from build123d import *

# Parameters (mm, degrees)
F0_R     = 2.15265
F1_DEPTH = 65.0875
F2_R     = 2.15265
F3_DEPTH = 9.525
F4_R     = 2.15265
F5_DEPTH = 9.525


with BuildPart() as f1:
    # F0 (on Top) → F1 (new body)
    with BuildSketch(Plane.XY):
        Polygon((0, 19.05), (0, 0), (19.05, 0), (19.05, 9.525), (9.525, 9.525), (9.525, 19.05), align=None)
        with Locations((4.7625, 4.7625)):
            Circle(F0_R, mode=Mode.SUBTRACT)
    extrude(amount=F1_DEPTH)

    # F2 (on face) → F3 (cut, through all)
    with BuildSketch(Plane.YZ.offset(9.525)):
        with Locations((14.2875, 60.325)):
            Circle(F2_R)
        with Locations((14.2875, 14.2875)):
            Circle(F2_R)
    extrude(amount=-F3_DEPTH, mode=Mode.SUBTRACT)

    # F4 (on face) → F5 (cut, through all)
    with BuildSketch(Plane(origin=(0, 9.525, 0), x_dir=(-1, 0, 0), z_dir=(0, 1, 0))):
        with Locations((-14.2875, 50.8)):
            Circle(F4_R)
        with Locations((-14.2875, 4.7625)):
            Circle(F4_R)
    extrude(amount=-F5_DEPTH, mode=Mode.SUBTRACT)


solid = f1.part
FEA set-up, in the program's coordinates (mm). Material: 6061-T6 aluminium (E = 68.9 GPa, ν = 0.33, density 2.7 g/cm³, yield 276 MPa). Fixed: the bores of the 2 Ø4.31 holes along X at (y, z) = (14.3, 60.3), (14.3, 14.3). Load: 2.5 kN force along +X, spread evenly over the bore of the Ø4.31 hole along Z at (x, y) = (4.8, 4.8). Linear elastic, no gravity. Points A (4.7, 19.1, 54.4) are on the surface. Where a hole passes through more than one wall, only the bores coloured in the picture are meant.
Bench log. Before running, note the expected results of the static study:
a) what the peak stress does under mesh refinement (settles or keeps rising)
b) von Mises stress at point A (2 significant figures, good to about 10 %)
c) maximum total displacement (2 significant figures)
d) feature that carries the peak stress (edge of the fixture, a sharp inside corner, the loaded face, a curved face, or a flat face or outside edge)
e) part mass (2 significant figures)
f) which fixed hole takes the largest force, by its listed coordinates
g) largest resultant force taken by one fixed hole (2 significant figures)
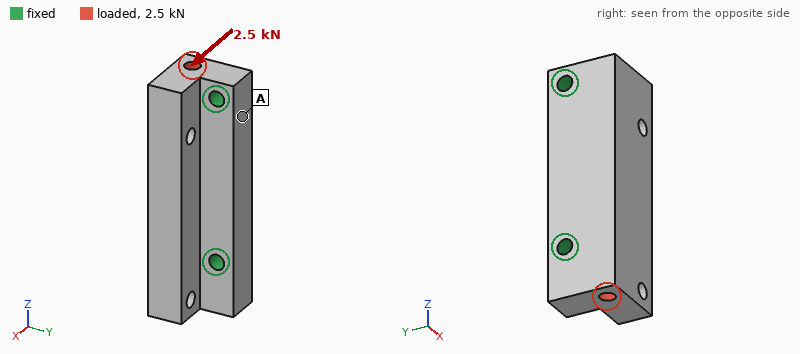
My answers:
keeps rising
15 MPa
23 µm
edge of the fixture
44 g
(14.3, 14.3)
1.5 kN
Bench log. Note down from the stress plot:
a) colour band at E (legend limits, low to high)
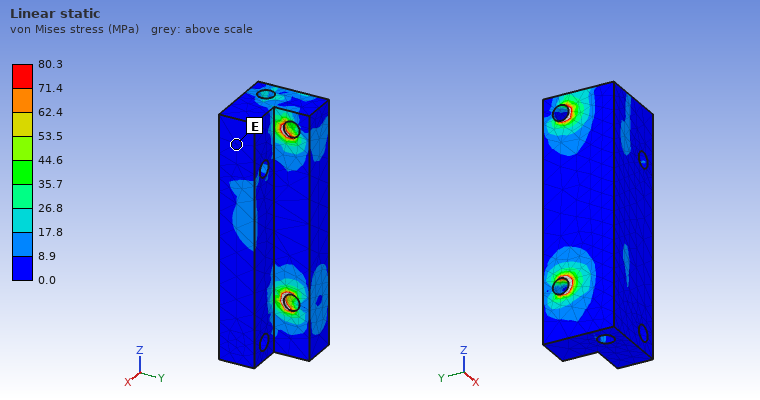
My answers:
0.0 to 8.9 MPa
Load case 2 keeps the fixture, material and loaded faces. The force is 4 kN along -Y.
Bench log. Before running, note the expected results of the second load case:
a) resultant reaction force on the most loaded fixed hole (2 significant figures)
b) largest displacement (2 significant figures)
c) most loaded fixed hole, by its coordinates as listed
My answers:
2.4 kN
7.8 µm
(14.3, 14.3)
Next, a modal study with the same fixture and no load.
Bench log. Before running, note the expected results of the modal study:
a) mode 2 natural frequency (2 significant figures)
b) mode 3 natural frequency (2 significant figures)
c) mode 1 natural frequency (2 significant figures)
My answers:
16 kHz
19 kHz
11 kHz
